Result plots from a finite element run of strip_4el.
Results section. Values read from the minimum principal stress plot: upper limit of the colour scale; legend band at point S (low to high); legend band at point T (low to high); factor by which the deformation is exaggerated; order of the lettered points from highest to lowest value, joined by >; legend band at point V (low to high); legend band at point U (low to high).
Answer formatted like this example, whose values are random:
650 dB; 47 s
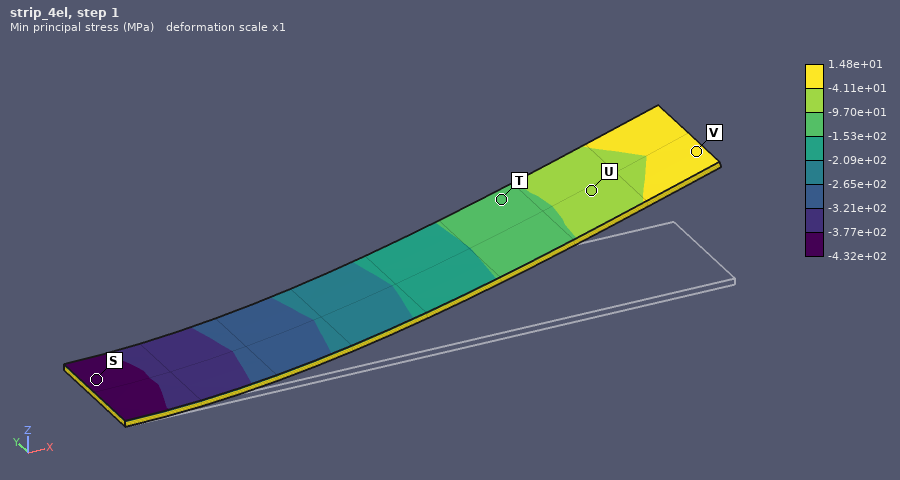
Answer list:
1.48e+01 MPa; -4.32e+02 to -3.77e+02 MPa; -1.53e+02 to -9.70e+01 MPa; 1; V > U > T > S; -4.11e+01 to 1.48e+01 MPa; -9.70e+01 to -4.11e+01 MPa
